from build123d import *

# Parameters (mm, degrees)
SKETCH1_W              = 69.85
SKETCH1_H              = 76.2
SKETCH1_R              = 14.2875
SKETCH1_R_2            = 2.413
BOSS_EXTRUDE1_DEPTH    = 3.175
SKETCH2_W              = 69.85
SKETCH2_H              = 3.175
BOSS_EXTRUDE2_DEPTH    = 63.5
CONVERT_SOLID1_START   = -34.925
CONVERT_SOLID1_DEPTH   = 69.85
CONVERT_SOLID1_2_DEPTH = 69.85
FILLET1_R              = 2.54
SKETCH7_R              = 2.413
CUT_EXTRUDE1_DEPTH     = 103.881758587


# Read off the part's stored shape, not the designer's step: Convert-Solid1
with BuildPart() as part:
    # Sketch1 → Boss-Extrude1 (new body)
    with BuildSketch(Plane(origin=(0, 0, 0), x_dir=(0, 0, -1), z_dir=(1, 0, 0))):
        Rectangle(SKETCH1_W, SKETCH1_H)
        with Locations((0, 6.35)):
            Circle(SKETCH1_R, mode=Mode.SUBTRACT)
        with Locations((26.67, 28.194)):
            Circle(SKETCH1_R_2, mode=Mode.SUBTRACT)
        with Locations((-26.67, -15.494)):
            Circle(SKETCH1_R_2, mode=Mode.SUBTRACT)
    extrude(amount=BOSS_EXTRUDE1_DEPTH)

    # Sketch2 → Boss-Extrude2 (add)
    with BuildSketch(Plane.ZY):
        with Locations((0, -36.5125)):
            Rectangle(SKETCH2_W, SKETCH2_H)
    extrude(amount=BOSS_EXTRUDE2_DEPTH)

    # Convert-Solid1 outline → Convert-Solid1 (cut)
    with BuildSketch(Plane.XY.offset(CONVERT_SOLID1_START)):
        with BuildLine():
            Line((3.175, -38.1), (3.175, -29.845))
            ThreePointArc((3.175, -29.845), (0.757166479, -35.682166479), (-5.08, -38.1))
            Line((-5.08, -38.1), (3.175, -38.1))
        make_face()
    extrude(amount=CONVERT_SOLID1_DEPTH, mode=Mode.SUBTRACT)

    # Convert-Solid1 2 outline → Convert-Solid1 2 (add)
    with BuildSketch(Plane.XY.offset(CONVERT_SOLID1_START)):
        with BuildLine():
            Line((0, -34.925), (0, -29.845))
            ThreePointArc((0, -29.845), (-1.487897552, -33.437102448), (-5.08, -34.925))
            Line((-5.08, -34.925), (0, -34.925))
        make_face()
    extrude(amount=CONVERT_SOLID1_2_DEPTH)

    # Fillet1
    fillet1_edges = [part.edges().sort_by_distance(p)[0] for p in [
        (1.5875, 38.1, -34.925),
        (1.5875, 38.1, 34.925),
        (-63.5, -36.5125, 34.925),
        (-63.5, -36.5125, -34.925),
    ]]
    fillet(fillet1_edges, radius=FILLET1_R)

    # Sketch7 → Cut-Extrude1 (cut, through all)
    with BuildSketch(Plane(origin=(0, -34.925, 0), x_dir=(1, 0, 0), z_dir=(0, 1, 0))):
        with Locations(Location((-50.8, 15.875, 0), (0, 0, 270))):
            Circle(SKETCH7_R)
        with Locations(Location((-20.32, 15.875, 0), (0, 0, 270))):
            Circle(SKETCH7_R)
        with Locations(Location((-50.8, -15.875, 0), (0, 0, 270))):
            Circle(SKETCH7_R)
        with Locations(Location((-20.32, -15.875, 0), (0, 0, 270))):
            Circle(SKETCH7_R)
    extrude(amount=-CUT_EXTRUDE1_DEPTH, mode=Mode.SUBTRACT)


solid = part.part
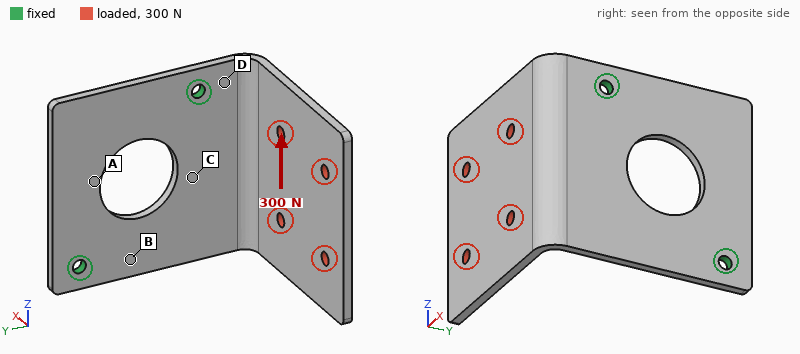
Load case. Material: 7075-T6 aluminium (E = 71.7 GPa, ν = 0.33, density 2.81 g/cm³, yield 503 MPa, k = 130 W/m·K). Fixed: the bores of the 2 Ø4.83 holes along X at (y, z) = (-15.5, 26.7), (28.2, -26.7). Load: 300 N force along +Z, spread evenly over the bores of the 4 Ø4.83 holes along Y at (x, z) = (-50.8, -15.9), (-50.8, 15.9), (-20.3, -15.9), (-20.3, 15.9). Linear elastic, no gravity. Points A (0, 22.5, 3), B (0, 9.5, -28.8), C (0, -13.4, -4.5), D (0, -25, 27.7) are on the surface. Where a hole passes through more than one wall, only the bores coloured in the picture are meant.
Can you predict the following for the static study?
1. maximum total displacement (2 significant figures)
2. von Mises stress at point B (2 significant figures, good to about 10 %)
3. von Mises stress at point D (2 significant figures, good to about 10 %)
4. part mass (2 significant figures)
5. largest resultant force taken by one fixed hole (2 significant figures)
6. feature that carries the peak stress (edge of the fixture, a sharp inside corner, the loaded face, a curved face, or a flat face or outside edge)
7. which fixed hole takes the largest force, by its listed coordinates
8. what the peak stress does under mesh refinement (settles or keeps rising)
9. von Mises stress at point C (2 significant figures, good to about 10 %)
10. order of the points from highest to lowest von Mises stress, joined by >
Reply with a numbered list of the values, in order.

1. 1.4 mm
2. 56 MPa
3. 110 MPa
4. 79 g
5. 310 N
6. edge of the fixture
7. (-15.5, 26.7)
8. keeps rising
9. 36 MPa
10. D > B > C > A
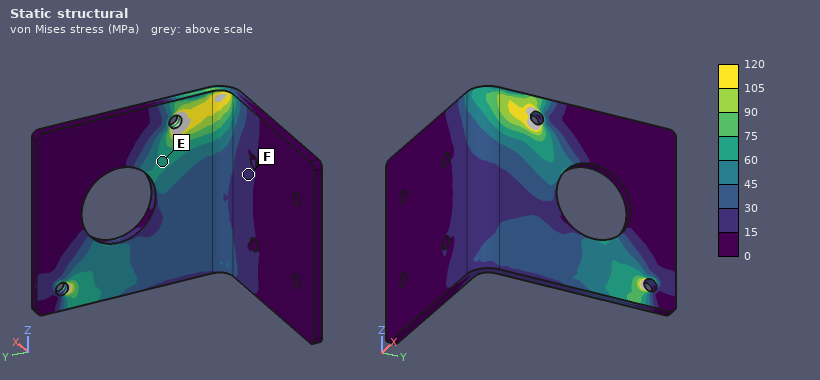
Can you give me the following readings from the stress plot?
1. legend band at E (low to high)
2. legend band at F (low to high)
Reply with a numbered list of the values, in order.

1. 60 to 75 MPa
2. 15 to 30 MPa
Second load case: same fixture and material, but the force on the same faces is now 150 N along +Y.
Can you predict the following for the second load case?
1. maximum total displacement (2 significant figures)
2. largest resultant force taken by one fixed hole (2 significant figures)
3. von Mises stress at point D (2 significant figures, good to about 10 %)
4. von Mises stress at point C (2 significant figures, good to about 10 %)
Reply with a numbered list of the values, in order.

1. 1.3 mm
2. 88 N
3. 71 MPa
4. 19 MPa
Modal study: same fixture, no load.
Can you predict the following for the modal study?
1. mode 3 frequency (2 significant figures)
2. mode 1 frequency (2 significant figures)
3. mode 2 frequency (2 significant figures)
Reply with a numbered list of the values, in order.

1. 1200 Hz
2. 330 Hz
3. 540 Hz
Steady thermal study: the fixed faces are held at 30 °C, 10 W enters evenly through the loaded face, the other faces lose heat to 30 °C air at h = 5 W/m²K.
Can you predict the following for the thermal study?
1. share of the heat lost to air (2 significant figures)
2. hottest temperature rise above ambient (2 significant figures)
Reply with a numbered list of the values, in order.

1. 12 %
2. 26 K
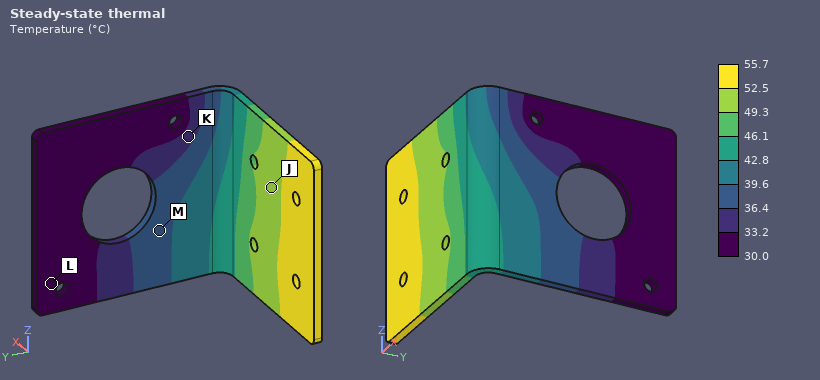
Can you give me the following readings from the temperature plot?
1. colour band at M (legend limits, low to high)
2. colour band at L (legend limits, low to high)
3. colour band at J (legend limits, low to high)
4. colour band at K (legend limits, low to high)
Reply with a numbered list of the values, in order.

1. 36.4 to 39.6 °C
2. 30.0 to 33.2 °C
3. 49.3 to 52.5 °C
4. 33.2 to 36.4 °C
